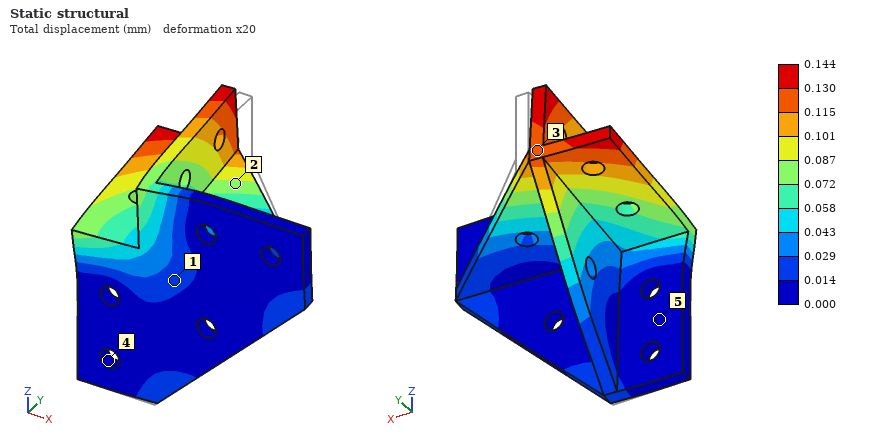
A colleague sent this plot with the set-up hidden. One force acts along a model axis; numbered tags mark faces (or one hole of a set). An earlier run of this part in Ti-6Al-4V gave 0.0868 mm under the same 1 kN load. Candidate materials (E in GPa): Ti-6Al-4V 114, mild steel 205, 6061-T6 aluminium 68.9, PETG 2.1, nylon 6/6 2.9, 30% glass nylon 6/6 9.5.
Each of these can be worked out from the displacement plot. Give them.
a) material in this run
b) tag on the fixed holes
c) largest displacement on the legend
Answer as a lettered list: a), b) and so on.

a) 6061-T6 aluminium
b) 4
c) 0.144 mm
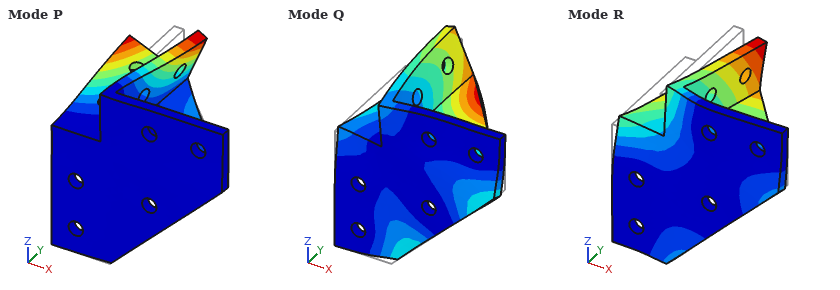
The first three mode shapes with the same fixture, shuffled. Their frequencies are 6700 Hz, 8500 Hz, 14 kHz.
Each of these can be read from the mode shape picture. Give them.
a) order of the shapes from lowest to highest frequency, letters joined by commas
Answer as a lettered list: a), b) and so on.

a) R, P, Q
